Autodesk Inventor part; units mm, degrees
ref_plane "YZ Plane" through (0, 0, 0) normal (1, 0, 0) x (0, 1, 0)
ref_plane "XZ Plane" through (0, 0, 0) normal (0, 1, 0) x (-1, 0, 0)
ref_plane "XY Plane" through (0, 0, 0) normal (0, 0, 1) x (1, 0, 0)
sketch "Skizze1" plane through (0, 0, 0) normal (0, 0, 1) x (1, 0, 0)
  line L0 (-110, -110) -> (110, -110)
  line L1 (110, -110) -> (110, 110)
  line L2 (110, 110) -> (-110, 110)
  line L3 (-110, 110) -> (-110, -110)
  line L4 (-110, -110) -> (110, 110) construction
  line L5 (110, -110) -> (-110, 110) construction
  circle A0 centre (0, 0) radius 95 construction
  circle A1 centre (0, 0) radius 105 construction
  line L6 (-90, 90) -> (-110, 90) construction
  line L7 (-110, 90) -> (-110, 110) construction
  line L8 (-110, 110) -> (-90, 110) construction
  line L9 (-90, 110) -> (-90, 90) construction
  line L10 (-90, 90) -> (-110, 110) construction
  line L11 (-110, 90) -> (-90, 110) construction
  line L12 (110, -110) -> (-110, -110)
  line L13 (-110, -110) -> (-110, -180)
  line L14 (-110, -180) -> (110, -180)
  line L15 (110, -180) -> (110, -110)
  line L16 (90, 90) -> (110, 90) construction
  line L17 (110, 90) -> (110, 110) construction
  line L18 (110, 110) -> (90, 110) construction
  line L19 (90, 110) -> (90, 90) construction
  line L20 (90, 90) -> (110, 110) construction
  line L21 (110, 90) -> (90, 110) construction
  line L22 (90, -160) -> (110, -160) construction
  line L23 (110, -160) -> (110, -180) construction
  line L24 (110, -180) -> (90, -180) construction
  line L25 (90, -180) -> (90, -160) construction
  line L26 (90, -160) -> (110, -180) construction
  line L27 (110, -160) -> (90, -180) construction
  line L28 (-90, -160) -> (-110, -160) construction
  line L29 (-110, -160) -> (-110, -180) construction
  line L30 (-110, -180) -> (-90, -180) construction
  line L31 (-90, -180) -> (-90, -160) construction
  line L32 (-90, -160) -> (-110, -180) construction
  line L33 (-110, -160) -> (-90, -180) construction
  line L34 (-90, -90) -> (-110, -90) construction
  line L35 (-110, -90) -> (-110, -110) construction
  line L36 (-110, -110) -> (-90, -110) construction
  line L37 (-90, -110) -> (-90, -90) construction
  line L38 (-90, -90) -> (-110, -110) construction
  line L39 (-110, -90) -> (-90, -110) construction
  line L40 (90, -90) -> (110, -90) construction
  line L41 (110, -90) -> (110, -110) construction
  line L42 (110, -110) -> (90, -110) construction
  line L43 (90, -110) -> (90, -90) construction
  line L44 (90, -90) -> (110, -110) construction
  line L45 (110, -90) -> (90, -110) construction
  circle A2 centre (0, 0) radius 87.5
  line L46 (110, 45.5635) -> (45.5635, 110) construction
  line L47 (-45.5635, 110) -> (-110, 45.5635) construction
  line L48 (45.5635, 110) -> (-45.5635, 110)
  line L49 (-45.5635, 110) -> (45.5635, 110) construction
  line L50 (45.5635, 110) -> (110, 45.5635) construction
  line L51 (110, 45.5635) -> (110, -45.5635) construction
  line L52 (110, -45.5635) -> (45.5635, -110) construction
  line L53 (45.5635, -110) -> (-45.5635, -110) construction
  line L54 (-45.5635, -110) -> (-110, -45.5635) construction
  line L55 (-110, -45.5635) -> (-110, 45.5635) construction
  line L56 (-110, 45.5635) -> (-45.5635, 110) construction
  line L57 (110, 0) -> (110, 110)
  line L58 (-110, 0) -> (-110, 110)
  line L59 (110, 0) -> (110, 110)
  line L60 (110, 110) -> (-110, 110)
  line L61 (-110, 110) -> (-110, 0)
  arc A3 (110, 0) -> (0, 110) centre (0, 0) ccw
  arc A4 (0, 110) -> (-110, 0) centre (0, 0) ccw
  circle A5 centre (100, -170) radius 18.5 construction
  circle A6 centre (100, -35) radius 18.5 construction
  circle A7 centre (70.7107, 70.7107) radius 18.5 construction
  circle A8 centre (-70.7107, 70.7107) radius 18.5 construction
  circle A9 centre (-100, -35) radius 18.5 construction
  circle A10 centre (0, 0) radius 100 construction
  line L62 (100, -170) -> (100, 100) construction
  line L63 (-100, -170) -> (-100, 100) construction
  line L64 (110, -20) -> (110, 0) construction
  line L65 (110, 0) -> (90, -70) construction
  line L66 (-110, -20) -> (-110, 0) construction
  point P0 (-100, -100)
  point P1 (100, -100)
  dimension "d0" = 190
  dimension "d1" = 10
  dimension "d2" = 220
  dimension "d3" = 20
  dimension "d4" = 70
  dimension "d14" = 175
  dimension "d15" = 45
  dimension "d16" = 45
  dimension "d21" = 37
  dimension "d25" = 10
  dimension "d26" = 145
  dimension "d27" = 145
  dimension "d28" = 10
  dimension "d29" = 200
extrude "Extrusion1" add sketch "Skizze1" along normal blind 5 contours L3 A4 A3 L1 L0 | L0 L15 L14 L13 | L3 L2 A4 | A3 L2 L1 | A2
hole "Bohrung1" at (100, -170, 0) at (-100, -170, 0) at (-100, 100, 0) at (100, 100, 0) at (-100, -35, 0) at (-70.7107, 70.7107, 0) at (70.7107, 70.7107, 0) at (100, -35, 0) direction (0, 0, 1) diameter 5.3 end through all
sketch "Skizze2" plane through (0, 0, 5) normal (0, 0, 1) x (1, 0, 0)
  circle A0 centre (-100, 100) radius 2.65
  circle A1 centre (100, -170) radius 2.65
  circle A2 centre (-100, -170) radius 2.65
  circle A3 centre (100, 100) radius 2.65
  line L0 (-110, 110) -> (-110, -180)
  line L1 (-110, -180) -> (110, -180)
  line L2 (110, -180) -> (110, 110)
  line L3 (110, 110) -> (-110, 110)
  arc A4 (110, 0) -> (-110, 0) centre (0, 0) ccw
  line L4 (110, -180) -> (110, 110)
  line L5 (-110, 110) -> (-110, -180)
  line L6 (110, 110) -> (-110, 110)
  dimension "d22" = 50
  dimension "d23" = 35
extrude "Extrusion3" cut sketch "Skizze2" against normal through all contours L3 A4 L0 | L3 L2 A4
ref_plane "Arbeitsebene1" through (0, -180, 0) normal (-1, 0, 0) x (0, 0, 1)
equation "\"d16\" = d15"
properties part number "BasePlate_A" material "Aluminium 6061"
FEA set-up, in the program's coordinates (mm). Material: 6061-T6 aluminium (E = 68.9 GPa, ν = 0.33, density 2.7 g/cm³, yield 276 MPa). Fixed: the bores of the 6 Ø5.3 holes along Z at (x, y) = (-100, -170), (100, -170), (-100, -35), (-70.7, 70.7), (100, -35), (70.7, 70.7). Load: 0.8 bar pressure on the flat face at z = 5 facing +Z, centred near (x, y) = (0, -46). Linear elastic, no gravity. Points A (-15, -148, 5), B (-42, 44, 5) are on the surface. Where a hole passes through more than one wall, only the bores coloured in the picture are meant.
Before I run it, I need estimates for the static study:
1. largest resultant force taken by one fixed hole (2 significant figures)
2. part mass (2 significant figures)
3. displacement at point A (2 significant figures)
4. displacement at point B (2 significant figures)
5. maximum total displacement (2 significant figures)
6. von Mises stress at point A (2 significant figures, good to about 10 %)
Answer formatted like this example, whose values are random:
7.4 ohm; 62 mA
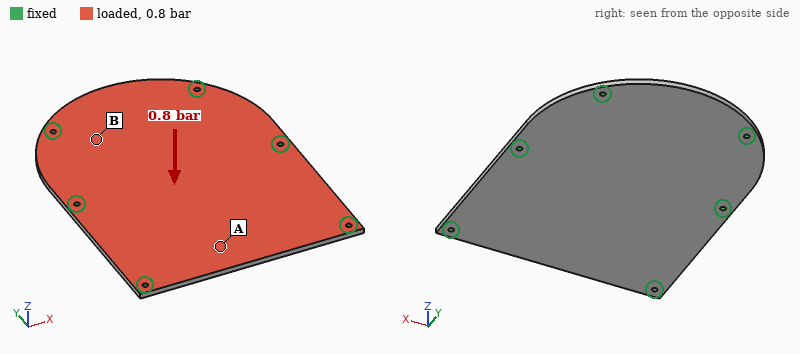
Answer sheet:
1.0 kN; 790 g; 0.73 mm; 0.20 mm; 0.79 mm; 37 MPa
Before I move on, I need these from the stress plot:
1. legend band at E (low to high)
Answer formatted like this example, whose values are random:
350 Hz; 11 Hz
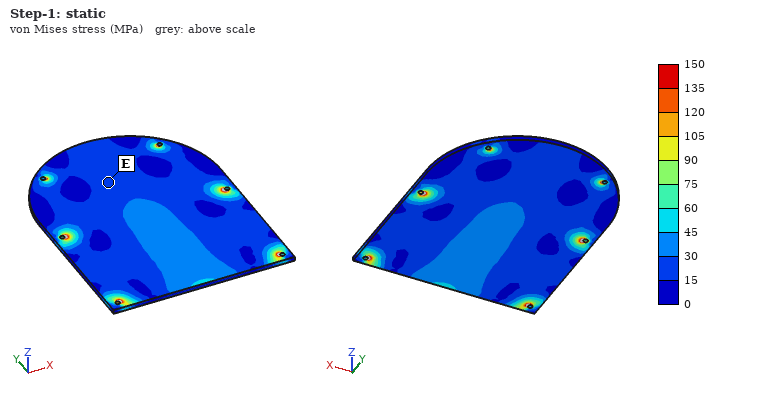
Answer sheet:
15 to 30 MPa
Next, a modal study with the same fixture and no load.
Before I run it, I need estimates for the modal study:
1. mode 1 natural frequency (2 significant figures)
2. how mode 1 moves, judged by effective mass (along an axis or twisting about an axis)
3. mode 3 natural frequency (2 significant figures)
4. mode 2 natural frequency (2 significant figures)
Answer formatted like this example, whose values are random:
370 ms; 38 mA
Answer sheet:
520 Hz; along Z; 1100 Hz; 820 Hz
